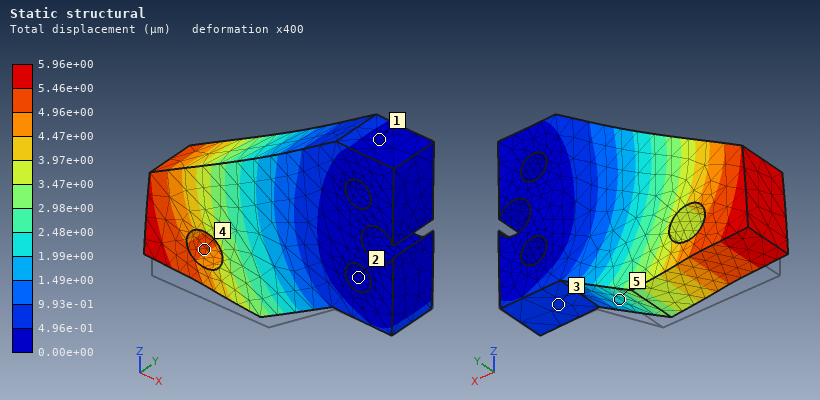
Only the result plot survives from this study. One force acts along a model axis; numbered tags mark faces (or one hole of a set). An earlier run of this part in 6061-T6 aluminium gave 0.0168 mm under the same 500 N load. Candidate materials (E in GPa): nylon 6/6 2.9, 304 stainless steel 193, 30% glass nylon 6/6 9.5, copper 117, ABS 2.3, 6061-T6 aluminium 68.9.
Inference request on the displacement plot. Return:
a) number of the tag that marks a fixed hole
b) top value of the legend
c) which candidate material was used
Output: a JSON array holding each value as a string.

["2", "5.96e+00 µm", "304 stainless steel"]
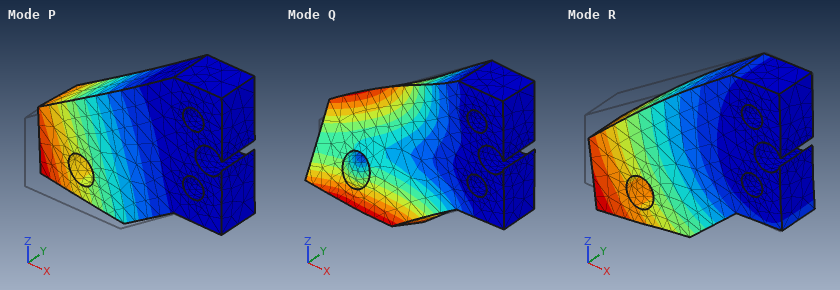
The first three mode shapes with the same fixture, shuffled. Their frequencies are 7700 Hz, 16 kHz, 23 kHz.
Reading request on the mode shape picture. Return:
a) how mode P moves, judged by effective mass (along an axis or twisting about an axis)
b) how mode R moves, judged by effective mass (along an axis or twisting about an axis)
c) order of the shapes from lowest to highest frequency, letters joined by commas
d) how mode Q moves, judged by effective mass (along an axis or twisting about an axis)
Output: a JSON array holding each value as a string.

["along Y", "along Z", "P, R, Q", "twisting about X"]
